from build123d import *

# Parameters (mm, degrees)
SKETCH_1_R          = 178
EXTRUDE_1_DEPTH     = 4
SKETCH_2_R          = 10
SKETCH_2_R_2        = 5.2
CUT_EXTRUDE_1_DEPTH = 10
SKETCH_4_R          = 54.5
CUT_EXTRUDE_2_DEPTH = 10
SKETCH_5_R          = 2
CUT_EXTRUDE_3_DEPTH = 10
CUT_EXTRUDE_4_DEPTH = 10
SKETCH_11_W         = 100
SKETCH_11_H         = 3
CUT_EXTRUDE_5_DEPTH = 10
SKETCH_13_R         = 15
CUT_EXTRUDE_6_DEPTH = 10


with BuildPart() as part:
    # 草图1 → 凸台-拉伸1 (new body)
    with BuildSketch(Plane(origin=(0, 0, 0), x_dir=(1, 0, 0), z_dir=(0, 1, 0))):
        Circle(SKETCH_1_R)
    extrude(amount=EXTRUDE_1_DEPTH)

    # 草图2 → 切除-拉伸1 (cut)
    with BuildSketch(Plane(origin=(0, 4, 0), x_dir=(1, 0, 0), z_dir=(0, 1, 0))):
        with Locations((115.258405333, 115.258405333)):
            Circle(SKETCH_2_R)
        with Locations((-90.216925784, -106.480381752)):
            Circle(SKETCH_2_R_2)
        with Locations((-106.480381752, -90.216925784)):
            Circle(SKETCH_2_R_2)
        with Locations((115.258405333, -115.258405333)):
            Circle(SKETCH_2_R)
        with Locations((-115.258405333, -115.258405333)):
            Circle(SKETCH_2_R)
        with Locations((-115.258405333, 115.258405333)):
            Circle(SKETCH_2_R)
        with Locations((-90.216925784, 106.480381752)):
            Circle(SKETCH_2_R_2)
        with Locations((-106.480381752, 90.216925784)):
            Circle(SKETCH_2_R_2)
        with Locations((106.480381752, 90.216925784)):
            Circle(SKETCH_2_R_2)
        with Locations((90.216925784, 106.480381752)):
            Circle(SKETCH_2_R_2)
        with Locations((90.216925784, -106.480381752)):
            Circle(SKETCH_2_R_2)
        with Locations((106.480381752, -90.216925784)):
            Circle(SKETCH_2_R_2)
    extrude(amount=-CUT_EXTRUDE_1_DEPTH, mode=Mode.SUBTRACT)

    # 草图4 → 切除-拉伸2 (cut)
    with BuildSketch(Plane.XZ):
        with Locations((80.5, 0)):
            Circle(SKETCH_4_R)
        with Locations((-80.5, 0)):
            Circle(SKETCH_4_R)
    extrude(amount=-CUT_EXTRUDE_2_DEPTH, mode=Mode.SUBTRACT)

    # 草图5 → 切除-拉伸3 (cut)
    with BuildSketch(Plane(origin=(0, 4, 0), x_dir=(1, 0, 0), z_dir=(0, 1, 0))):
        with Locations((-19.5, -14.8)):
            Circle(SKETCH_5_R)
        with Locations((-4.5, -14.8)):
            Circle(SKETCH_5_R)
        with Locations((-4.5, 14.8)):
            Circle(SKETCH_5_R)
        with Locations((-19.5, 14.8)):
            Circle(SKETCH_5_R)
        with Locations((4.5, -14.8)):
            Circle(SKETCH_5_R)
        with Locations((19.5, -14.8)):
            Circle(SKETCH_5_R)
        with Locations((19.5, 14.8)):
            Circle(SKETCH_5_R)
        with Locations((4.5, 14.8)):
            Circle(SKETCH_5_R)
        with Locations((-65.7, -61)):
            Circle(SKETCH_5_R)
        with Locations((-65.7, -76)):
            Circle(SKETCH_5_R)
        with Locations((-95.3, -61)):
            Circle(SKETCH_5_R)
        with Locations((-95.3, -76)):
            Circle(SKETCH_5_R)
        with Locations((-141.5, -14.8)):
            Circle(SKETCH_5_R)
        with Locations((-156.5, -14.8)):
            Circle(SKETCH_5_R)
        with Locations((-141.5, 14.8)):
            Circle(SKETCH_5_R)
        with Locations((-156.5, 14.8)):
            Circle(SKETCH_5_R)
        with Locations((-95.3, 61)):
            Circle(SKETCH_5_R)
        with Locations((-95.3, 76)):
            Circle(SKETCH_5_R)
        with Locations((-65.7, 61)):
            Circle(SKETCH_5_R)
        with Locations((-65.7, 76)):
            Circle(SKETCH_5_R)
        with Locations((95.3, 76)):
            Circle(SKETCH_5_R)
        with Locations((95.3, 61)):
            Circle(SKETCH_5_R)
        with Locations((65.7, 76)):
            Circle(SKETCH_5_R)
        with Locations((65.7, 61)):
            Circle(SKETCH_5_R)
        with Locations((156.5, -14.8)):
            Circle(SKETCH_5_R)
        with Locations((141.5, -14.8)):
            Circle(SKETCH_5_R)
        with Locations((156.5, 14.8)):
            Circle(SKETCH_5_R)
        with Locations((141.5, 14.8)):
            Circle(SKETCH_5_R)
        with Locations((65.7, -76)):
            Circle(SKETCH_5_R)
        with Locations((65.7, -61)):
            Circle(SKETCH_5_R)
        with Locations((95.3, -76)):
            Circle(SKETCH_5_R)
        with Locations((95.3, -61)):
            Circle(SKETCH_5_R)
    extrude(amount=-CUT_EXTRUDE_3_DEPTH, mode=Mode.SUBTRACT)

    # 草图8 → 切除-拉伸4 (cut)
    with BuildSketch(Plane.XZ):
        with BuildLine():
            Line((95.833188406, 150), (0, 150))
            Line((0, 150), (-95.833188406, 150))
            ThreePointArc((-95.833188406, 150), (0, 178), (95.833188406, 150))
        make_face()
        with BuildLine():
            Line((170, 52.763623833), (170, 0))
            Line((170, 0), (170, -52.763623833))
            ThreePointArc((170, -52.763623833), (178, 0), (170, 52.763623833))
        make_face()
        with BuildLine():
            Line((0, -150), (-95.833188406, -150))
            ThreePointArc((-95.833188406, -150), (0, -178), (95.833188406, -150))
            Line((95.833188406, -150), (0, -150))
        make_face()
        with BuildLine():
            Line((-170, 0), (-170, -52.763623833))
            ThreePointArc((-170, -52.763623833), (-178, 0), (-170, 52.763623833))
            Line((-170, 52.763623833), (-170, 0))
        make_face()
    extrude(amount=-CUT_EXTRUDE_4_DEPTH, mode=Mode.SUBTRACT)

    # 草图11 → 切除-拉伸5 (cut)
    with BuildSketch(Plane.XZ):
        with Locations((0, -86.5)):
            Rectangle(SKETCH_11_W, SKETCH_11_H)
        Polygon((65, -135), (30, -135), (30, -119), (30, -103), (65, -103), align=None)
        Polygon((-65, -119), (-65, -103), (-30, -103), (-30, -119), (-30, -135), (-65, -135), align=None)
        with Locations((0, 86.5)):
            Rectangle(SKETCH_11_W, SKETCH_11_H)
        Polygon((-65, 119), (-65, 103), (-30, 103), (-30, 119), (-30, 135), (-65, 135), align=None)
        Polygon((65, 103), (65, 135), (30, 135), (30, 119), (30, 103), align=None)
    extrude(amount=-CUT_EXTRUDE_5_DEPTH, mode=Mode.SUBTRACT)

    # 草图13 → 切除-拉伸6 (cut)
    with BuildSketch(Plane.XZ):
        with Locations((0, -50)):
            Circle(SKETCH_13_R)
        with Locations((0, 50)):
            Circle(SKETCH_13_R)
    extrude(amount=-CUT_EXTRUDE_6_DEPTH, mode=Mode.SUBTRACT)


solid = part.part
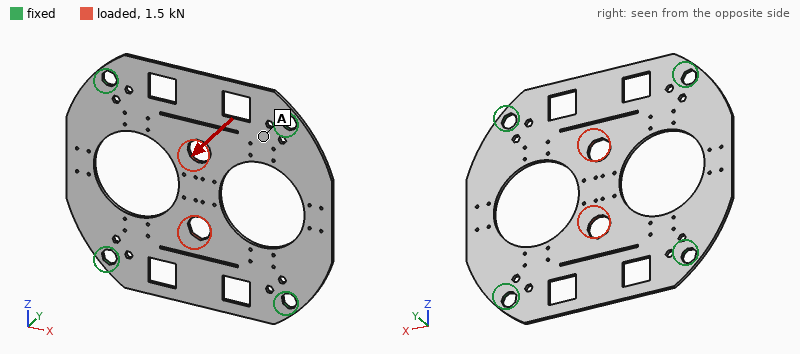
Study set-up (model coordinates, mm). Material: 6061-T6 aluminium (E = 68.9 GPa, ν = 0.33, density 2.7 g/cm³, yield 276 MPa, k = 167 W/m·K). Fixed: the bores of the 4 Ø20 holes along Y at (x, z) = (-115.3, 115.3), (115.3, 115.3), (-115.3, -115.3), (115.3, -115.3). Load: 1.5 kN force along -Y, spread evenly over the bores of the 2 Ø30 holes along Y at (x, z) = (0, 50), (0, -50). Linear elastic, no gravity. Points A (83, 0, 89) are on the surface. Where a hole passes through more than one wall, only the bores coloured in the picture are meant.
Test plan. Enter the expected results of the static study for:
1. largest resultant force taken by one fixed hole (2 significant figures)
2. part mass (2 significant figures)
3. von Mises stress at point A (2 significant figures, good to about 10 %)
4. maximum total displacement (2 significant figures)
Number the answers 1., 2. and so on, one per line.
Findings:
1. 380 N
2. 690 g
3. 52 MPa
4. 3.4 mm
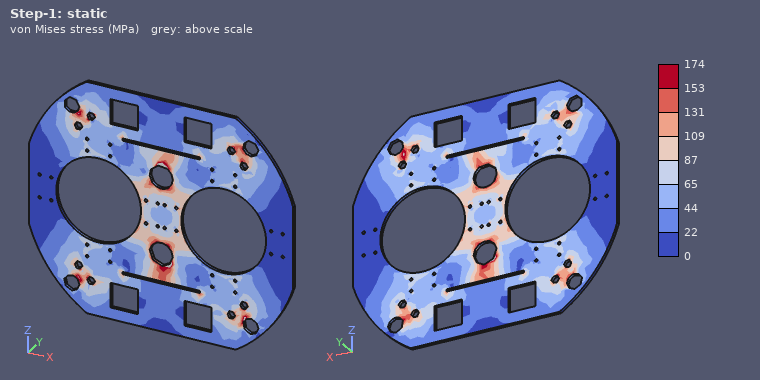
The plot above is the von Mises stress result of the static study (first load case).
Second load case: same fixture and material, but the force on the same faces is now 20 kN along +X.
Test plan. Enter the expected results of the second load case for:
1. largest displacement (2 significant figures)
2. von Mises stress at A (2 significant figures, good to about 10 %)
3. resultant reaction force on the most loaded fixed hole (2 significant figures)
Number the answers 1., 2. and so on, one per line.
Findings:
1. 79 µm
2. 31 MPa
3. 5.2 kN
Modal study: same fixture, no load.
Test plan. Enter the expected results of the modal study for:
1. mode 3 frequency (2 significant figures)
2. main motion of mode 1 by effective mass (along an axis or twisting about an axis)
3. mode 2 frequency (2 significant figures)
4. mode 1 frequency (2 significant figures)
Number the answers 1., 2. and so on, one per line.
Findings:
1. 420 Hz
2. along Y
3. 410 Hz
4. 300 Hz
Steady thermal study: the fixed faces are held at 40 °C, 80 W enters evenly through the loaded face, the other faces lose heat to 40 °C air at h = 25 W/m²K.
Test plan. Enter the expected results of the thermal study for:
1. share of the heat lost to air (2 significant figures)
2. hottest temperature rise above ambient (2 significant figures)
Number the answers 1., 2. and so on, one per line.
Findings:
1. 54 %
2. 49 K
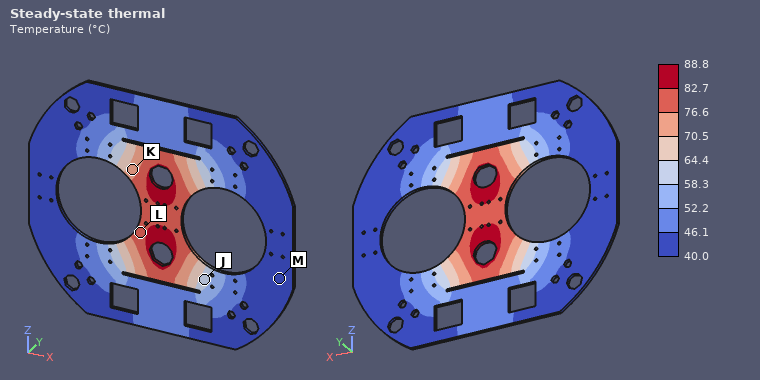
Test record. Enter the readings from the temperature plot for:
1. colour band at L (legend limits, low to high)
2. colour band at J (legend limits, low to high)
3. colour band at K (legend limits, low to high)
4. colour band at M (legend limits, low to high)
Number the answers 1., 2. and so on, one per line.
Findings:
1. 76.6 to 82.7 °C
2. 58.3 to 64.4 °C
3. 70.5 to 76.6 °C
4. 40.0 to 46.1 °C
